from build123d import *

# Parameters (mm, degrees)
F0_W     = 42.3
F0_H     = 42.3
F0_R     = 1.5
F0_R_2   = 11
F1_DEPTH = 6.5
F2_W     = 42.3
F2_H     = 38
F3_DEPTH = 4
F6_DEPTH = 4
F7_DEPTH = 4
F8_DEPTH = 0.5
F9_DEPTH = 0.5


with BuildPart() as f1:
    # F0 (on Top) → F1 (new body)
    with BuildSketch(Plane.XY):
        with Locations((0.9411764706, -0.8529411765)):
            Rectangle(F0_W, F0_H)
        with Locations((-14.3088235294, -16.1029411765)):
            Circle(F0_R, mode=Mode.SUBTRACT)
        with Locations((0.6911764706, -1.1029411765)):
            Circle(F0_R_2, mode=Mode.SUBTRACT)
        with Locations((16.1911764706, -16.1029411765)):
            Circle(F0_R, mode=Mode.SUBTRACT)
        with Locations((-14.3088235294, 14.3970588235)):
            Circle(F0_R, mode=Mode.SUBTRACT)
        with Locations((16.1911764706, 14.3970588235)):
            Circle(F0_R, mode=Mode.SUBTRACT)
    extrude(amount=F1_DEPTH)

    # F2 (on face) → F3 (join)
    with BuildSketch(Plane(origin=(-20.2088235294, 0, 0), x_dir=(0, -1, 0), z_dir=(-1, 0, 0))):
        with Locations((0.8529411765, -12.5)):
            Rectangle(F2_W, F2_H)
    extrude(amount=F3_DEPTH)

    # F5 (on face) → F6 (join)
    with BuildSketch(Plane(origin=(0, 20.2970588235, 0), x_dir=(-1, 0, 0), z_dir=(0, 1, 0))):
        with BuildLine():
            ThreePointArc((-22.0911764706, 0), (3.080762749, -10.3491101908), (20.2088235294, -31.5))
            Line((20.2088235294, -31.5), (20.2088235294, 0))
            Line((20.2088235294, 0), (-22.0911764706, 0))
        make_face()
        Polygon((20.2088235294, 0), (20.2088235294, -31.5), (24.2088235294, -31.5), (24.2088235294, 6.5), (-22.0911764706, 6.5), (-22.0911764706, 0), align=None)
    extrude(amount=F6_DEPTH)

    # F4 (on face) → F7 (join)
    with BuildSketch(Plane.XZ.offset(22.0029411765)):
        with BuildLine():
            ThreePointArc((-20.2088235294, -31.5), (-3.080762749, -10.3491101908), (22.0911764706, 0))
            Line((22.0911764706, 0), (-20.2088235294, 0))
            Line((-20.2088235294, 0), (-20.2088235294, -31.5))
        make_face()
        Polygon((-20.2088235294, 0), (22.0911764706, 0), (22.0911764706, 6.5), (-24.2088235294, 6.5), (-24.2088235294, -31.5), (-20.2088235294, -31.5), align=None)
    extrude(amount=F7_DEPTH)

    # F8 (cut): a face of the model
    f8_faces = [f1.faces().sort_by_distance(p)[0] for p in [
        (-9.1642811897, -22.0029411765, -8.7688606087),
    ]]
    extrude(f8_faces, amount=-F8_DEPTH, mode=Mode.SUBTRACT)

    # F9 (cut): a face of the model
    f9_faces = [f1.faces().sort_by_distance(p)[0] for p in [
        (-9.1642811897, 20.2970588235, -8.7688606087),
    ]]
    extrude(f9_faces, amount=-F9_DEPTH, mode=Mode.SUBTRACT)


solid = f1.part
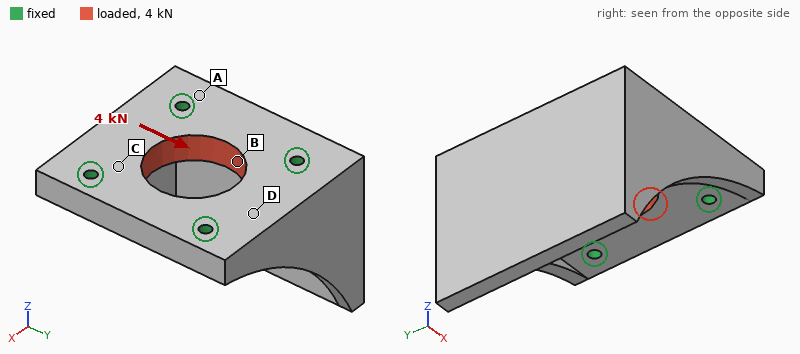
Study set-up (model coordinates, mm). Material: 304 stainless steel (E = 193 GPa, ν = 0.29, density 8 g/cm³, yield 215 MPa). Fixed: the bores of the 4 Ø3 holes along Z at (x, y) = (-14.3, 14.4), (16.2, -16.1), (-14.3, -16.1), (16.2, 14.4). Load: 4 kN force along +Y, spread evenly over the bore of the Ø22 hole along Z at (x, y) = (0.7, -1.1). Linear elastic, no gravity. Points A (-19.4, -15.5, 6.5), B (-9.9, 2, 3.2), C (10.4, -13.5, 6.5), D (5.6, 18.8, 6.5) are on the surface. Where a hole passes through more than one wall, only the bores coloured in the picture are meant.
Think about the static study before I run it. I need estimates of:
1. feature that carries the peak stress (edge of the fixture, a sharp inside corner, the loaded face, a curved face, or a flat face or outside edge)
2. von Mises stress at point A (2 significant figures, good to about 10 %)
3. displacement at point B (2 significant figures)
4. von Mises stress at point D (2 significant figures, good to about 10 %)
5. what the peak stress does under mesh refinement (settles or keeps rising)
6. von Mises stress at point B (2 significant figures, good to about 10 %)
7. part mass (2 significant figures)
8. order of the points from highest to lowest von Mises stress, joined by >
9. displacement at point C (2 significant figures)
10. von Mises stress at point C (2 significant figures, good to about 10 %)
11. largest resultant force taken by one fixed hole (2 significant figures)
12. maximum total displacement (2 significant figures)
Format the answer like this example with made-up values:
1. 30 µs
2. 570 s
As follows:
1. edge of the fixture
2. 2.7 MPa
3. 0.82 µm
4. 6.5 MPa
5. keeps rising
6. 15 MPa
7. 170 g
8. B > C > D > A
9. 0.71 µm
10. 9.7 MPa
11. 1.0 kN
12. 1.5 µm
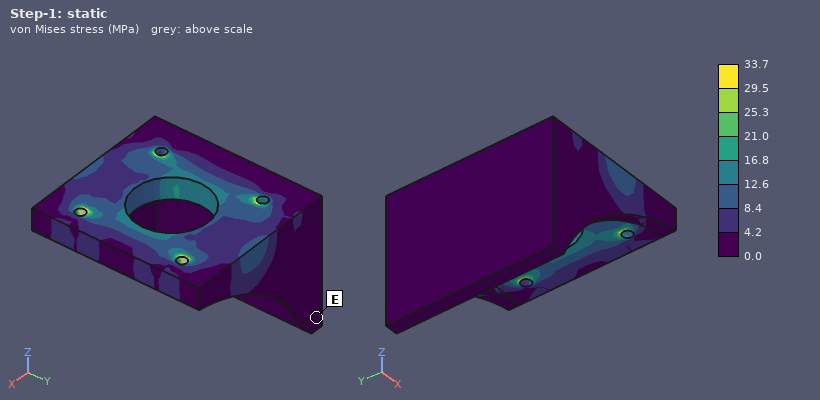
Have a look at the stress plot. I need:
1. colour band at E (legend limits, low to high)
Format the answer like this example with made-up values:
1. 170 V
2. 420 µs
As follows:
1. 0.0 to 4.2 MPa
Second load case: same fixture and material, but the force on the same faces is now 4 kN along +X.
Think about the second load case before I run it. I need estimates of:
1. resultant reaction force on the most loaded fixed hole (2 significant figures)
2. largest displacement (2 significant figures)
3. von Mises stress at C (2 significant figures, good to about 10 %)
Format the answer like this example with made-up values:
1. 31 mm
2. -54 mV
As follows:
1. 1.0 kN
2. 1.9 µm
3. 14 MPa
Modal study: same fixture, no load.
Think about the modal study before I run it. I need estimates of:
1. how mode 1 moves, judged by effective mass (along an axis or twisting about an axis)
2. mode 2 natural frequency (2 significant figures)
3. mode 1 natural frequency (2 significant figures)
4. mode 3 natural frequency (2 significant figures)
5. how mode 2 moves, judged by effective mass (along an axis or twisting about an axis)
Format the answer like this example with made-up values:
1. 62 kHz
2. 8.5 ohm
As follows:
1. along X
2. 8300 Hz
3. 5500 Hz
4. 12 kHz
5. along Y
